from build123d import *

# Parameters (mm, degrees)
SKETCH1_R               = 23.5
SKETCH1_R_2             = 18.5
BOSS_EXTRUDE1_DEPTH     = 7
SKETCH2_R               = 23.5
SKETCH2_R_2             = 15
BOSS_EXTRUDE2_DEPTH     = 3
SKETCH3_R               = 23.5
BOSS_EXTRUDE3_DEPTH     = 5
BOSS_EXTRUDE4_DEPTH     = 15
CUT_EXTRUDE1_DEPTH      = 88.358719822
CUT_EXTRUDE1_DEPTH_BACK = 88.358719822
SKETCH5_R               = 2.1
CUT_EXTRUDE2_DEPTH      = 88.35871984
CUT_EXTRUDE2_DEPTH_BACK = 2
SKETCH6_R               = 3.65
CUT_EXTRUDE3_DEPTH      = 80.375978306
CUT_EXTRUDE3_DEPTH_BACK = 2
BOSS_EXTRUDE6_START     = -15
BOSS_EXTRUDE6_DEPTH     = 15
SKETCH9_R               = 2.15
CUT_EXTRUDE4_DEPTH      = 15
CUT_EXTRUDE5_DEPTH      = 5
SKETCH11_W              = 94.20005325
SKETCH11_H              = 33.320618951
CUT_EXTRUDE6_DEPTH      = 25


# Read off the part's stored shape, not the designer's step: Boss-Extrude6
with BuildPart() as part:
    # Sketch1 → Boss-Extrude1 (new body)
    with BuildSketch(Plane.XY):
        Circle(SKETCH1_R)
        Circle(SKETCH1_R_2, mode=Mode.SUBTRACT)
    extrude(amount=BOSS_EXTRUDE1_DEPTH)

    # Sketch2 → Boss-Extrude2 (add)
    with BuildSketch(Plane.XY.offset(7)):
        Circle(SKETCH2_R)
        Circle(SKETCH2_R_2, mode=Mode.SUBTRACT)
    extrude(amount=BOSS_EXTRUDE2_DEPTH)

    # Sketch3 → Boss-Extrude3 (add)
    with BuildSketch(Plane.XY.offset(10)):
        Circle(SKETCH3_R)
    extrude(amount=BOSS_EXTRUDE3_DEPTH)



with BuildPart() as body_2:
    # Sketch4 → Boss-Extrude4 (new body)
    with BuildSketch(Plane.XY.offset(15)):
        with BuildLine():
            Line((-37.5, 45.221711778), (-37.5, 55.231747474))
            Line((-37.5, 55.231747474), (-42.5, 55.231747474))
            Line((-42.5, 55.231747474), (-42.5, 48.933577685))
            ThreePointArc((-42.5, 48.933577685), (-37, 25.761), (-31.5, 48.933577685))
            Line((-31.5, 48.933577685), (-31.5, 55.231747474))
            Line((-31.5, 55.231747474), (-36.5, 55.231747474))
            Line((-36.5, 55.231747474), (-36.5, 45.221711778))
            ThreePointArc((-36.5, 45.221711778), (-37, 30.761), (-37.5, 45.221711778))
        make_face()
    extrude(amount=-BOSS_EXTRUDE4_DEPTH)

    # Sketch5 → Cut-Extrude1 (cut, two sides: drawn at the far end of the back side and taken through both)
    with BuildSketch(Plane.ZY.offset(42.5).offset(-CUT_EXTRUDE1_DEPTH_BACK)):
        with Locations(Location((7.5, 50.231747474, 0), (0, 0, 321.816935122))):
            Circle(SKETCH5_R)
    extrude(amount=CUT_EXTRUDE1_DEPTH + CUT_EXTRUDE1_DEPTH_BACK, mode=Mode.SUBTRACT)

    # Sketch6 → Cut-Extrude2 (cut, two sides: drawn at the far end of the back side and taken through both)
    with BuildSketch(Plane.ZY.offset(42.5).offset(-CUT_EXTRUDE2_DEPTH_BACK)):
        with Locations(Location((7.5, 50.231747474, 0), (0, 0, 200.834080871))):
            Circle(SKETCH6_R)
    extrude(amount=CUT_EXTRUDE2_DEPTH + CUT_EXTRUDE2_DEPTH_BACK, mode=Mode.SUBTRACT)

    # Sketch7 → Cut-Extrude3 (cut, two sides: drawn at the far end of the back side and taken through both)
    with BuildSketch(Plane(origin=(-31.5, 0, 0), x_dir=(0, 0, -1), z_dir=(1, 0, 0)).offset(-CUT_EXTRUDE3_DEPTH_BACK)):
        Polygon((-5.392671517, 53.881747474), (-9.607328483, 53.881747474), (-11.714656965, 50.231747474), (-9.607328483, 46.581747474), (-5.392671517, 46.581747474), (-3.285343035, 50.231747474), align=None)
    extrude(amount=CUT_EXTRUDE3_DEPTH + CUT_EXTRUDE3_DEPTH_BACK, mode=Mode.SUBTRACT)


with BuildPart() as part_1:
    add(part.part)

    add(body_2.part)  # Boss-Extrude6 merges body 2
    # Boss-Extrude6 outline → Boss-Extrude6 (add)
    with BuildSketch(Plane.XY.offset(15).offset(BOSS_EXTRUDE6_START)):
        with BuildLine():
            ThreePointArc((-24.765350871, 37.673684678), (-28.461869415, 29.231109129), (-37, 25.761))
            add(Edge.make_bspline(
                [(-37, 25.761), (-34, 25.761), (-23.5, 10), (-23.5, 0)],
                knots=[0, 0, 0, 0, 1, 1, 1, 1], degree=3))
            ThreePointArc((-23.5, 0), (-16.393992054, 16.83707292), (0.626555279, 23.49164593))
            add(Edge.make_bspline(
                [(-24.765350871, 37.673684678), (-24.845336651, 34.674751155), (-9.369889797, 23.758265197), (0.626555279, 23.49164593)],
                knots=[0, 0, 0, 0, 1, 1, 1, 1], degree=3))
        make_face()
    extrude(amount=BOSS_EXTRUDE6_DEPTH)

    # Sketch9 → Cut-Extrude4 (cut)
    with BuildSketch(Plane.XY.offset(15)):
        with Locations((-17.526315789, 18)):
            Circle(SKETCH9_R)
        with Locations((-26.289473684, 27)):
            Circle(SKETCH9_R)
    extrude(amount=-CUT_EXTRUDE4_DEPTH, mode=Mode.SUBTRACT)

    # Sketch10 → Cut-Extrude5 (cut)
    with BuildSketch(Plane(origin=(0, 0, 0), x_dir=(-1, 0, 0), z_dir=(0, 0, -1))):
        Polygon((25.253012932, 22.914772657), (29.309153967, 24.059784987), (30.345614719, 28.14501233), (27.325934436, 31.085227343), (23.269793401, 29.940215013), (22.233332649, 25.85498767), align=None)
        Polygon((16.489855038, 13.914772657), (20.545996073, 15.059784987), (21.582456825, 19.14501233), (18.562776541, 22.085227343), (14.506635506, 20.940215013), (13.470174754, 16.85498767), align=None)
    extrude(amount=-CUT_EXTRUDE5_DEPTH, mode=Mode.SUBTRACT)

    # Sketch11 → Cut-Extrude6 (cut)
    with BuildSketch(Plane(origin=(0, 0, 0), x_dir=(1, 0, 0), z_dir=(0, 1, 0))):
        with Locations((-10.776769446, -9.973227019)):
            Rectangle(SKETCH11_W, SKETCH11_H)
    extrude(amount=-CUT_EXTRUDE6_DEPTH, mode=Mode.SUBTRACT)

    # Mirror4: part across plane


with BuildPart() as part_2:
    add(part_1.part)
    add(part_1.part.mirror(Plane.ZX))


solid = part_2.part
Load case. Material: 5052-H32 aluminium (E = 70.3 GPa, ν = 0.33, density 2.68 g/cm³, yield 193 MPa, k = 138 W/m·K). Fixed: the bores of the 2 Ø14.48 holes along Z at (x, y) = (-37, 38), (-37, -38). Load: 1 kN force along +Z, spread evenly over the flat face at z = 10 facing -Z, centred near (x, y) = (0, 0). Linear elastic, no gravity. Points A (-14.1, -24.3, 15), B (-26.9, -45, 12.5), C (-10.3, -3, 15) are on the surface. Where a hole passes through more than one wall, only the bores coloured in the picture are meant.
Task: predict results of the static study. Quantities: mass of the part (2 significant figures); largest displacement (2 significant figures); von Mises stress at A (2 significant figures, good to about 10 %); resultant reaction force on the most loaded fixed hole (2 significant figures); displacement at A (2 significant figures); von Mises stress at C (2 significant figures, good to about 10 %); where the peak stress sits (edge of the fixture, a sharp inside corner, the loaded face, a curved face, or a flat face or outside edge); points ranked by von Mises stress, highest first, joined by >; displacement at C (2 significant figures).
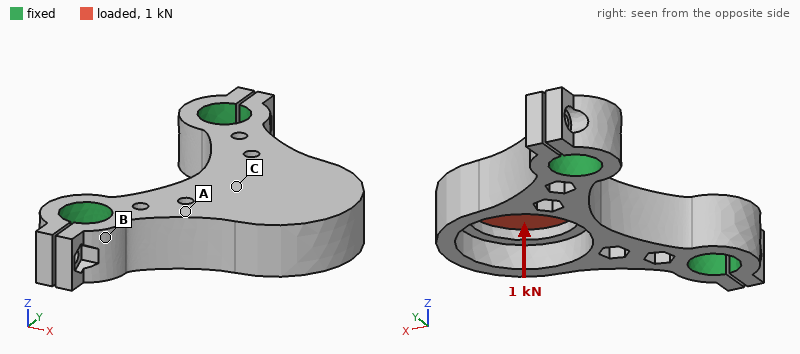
98 g
86 µm
17 MPa
500 N
19 µm
8.5 MPa
a curved face
A > C > B
31 µm
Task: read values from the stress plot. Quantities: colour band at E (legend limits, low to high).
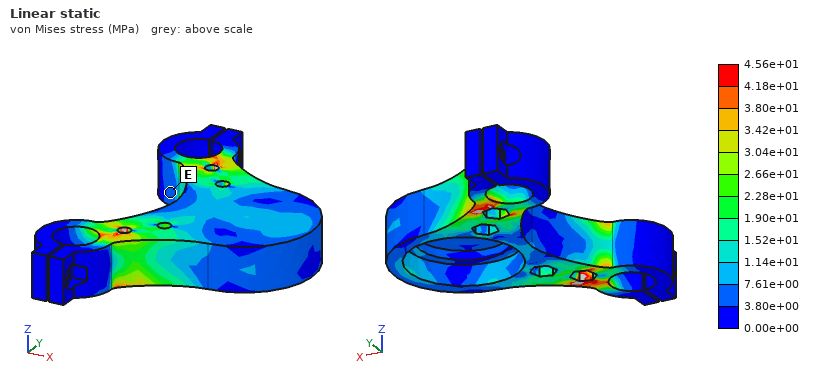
3.80e+00 to 7.61e+00 MPa
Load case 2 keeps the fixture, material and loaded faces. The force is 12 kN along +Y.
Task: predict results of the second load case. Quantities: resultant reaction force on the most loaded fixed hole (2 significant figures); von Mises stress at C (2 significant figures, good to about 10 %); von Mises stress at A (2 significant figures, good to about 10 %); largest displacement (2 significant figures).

8.1 kN
47 MPa
56 MPa
81 µm
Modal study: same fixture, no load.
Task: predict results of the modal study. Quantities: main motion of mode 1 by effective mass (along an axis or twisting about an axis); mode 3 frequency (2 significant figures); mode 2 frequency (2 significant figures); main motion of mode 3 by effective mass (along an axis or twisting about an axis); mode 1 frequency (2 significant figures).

along Z
12 kHz
7800 Hz
along Z
3200 Hz
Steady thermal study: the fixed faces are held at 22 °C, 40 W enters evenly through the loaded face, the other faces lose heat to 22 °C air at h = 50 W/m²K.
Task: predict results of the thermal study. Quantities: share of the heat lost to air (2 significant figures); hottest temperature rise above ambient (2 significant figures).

17 %
26 K
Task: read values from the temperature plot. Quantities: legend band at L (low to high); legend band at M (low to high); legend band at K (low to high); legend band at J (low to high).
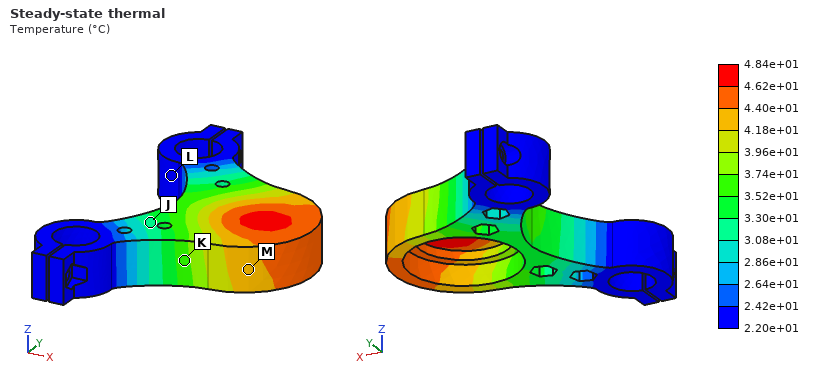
2.20e+01 to 2.42e+01 °C
4.18e+01 to 4.40e+01 °C
3.52e+01 to 3.74e+01 °C
3.08e+01 to 3.30e+01 °C
